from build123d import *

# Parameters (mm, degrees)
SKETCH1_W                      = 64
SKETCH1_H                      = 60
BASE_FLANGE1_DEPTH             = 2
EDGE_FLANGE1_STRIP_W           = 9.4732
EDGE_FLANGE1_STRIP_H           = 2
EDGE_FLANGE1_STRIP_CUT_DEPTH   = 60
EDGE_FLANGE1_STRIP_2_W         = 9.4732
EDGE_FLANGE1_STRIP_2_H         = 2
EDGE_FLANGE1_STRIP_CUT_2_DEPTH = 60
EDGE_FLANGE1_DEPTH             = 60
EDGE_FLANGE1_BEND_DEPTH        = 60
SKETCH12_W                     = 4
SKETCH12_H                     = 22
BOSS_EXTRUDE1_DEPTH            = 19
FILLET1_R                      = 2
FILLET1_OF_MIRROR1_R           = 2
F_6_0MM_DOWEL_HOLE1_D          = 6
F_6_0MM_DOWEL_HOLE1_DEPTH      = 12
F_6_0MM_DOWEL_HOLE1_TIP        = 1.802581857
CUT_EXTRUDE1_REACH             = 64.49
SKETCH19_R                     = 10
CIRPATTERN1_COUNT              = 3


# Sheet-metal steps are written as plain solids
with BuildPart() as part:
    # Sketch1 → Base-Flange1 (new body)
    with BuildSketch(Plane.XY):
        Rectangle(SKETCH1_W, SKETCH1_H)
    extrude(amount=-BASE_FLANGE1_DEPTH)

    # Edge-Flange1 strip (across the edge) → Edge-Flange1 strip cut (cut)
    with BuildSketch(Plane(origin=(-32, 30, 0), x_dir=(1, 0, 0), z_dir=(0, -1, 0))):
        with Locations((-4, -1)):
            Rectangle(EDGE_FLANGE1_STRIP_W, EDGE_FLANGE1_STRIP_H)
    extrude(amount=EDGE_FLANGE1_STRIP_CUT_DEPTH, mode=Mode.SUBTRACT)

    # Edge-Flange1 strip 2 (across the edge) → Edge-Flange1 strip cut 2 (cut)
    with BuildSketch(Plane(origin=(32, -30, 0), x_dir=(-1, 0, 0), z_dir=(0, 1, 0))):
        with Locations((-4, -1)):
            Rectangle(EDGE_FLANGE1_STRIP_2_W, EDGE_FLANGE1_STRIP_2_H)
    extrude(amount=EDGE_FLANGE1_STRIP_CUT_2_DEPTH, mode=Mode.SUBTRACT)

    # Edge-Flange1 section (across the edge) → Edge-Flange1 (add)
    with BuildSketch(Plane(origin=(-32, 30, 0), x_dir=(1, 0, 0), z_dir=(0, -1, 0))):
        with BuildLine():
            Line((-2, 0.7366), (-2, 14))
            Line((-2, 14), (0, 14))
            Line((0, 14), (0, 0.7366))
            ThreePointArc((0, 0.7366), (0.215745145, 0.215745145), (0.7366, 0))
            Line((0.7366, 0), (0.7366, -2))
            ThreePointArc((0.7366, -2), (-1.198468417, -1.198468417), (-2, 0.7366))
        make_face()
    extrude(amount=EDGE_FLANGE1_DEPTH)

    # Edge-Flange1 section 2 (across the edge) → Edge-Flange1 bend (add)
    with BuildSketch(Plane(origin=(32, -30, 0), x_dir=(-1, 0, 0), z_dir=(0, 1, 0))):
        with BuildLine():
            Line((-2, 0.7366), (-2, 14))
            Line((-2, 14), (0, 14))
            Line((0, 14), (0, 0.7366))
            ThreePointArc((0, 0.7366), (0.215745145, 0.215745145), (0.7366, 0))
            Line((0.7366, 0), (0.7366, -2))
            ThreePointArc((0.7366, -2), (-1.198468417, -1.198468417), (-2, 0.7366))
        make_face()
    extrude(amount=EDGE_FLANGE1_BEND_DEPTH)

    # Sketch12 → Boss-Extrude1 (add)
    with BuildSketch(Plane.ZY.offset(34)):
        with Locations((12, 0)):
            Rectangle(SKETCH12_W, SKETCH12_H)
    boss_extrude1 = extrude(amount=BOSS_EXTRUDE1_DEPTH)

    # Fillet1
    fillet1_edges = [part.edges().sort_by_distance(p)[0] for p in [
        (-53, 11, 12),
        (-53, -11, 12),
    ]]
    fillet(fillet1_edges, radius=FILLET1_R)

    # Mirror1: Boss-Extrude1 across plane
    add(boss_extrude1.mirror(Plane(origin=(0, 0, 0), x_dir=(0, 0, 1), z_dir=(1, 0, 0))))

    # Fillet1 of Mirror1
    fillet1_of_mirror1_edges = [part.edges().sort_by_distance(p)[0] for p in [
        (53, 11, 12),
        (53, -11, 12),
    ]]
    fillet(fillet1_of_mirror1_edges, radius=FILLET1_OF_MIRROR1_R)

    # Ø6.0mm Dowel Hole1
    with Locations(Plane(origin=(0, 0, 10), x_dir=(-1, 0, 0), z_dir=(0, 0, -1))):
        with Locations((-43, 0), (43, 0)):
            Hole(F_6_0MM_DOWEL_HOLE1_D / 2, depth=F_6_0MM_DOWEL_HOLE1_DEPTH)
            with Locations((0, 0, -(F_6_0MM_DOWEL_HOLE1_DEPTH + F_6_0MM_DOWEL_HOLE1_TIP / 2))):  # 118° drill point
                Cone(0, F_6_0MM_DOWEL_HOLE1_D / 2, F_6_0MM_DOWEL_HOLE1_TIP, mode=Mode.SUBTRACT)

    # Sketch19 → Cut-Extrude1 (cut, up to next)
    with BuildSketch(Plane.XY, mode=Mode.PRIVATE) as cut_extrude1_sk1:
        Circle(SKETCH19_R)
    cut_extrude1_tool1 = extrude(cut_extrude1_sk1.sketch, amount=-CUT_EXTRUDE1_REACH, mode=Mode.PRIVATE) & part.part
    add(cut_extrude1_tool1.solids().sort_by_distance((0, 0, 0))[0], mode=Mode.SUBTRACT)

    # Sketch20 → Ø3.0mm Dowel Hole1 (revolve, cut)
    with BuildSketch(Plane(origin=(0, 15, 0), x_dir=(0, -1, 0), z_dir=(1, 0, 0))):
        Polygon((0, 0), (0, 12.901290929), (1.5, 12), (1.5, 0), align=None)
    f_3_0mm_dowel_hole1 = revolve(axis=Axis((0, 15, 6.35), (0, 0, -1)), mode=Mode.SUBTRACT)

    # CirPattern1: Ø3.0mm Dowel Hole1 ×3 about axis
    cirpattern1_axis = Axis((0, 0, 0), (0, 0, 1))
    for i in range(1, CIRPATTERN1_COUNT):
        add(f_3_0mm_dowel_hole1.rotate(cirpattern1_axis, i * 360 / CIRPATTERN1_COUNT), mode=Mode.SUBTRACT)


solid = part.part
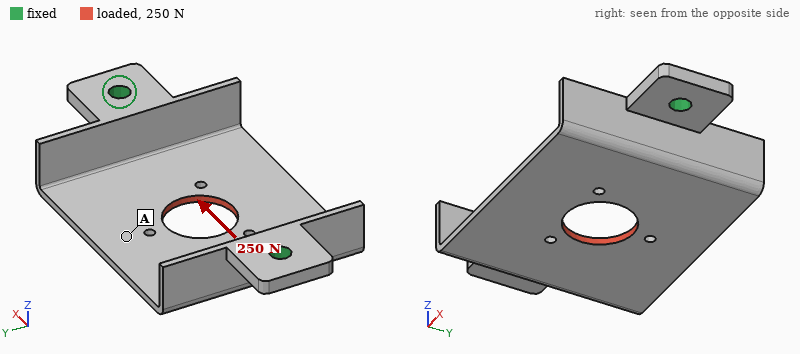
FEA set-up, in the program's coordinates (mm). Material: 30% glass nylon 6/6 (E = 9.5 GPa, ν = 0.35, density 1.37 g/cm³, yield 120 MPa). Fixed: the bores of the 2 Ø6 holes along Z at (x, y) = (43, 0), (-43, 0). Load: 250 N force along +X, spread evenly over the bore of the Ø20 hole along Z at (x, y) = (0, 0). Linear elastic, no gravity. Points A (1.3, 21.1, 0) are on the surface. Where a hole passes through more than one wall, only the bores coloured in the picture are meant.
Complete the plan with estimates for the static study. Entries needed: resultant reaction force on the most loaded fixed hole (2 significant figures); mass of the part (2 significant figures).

130 N
19 g
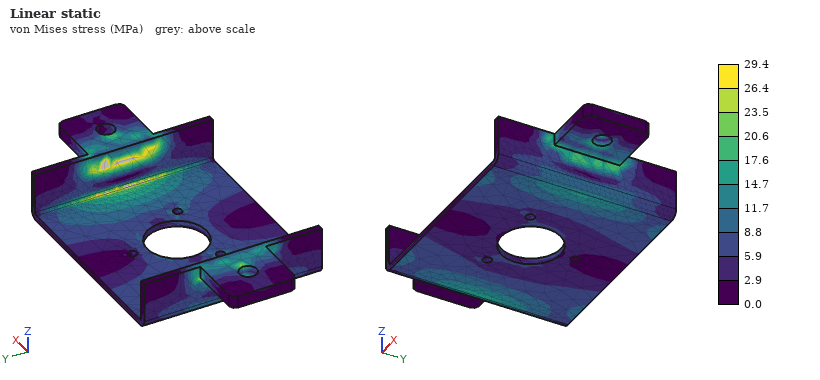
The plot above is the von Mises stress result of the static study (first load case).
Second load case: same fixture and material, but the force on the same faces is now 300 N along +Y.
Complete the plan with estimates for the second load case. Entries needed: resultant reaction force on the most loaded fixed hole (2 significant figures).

150 N
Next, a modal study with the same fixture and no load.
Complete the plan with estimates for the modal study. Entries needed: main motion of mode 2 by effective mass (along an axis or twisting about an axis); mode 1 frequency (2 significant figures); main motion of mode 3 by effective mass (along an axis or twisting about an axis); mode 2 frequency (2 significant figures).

along Z
1000 Hz
along X
1100 Hz
